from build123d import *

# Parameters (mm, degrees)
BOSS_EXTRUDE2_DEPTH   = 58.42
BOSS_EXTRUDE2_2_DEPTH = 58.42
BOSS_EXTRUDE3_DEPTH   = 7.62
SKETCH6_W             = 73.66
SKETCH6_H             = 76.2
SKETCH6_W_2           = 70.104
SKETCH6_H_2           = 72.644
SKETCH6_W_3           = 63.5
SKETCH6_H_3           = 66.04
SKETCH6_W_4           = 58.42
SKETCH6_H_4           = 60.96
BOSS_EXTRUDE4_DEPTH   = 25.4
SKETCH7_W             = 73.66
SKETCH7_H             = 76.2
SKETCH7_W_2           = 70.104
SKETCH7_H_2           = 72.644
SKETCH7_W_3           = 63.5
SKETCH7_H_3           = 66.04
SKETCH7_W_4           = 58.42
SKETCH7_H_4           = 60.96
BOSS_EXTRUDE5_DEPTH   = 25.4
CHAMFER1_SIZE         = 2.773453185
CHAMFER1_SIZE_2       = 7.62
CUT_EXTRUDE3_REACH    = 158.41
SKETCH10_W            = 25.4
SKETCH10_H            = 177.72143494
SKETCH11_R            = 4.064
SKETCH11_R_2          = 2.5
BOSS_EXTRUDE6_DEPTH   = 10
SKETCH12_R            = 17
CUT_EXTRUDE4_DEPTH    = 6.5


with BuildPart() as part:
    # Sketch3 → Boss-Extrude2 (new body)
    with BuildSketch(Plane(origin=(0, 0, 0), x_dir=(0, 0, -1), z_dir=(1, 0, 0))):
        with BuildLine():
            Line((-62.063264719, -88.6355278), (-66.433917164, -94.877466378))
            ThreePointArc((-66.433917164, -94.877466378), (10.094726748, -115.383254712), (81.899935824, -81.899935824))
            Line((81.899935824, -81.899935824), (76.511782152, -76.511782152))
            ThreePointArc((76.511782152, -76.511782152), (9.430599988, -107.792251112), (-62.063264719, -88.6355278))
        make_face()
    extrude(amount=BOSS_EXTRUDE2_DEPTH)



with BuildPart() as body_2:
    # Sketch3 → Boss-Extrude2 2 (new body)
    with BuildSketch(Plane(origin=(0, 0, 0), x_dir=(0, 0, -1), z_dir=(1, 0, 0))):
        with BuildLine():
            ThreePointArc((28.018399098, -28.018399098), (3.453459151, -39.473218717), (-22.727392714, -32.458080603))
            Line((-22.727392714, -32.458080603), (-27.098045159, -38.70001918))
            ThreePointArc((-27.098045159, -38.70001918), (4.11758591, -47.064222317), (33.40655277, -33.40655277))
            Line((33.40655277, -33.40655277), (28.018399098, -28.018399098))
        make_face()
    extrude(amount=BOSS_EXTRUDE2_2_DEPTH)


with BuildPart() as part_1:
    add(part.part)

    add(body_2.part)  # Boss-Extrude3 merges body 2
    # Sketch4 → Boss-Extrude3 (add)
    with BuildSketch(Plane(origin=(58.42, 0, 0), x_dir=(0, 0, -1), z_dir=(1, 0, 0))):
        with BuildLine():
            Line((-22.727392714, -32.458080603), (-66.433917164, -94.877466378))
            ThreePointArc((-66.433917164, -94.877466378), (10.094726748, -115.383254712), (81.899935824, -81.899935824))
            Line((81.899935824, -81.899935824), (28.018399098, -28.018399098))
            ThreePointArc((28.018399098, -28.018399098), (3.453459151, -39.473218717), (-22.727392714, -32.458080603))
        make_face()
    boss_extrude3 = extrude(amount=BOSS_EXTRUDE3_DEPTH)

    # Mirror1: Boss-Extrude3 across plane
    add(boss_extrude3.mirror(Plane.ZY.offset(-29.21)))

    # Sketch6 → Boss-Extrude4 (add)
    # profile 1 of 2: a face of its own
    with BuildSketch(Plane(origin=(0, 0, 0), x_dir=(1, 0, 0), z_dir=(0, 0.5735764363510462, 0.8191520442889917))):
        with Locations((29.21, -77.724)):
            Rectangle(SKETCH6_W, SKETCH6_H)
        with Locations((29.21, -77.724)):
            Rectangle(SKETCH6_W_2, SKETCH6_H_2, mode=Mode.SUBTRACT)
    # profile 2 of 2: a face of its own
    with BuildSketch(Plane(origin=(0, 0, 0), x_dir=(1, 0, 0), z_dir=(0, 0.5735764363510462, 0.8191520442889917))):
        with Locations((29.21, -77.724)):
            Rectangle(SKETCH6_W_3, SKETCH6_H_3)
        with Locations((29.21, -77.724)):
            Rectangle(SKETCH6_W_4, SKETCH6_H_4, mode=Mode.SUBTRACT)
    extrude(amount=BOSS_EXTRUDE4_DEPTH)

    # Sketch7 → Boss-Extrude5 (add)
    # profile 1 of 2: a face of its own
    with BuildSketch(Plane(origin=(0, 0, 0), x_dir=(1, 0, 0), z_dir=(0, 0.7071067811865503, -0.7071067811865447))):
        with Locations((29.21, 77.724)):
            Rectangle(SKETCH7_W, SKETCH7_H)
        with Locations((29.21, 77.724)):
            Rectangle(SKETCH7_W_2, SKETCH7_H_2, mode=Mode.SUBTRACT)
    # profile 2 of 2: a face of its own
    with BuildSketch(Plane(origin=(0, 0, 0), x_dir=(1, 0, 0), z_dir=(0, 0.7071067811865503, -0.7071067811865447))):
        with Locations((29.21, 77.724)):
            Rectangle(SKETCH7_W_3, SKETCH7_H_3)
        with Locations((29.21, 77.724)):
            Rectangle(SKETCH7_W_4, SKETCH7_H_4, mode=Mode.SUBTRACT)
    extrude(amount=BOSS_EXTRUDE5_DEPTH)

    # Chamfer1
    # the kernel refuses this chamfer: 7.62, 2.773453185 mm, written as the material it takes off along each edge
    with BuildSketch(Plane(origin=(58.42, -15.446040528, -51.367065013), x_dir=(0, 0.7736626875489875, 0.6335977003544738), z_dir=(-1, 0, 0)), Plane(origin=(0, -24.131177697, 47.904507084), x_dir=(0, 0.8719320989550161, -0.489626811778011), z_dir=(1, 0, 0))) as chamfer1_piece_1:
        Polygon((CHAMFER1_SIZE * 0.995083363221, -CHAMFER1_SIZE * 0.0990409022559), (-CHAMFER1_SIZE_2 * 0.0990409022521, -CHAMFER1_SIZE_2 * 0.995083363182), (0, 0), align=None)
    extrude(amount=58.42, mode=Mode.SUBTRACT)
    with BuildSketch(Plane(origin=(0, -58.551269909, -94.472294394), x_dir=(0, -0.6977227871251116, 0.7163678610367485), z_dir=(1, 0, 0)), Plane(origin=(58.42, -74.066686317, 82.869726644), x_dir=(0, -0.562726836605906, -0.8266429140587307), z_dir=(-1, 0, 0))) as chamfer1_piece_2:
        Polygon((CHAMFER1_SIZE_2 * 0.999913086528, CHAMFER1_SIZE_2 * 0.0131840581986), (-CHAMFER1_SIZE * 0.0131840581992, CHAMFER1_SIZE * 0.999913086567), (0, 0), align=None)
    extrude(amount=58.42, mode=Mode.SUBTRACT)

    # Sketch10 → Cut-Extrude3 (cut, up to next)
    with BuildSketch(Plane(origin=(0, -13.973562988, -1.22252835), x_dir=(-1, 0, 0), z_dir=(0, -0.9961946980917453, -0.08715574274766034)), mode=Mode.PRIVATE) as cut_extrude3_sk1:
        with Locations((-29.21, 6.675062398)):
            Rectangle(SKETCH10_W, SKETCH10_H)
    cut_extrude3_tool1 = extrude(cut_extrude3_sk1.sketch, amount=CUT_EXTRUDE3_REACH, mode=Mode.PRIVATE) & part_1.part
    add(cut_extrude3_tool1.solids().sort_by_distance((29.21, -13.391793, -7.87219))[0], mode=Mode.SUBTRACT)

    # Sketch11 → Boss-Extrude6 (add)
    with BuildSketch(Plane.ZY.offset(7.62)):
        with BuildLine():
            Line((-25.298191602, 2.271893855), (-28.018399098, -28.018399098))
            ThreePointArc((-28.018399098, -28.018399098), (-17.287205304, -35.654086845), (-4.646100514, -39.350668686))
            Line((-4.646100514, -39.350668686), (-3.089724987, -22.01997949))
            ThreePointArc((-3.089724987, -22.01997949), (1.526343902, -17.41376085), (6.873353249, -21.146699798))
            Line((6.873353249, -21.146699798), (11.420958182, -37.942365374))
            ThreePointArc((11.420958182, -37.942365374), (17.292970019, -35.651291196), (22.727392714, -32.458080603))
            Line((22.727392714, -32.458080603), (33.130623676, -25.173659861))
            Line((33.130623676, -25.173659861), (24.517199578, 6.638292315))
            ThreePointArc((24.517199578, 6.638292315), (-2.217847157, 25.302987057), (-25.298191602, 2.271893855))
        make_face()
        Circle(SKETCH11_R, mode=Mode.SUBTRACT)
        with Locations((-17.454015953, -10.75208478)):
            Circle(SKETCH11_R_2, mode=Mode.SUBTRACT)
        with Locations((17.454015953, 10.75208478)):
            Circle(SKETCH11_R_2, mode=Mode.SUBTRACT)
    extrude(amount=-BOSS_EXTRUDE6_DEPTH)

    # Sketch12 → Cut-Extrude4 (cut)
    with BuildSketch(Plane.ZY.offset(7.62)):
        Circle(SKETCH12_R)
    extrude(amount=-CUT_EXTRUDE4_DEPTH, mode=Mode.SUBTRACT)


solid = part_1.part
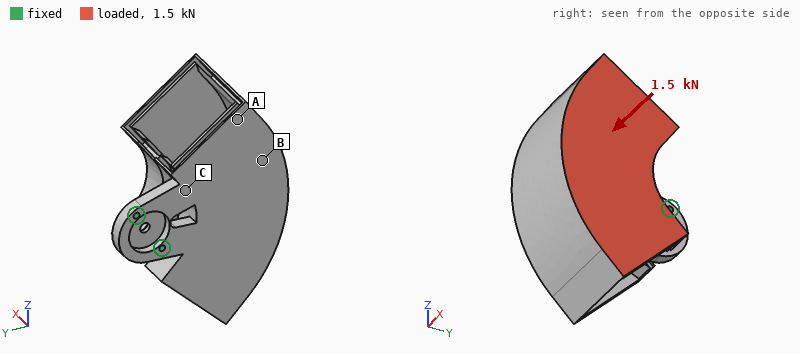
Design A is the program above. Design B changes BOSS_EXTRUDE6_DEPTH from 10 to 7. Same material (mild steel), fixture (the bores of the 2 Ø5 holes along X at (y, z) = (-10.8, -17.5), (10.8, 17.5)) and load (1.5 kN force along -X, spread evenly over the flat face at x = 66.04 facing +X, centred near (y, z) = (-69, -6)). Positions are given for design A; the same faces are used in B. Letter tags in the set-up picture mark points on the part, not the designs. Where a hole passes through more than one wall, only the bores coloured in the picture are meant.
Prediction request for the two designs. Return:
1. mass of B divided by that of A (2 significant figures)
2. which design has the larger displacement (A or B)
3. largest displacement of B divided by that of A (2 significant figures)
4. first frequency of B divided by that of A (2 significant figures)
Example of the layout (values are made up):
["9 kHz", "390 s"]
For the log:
["0.97", "B", "2.8", "0.67"]
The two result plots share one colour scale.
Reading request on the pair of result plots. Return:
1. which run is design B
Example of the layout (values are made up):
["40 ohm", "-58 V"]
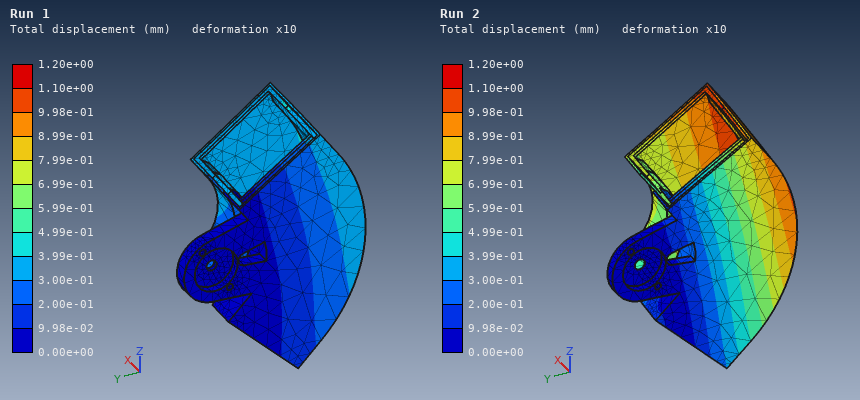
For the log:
["Run 2"]
